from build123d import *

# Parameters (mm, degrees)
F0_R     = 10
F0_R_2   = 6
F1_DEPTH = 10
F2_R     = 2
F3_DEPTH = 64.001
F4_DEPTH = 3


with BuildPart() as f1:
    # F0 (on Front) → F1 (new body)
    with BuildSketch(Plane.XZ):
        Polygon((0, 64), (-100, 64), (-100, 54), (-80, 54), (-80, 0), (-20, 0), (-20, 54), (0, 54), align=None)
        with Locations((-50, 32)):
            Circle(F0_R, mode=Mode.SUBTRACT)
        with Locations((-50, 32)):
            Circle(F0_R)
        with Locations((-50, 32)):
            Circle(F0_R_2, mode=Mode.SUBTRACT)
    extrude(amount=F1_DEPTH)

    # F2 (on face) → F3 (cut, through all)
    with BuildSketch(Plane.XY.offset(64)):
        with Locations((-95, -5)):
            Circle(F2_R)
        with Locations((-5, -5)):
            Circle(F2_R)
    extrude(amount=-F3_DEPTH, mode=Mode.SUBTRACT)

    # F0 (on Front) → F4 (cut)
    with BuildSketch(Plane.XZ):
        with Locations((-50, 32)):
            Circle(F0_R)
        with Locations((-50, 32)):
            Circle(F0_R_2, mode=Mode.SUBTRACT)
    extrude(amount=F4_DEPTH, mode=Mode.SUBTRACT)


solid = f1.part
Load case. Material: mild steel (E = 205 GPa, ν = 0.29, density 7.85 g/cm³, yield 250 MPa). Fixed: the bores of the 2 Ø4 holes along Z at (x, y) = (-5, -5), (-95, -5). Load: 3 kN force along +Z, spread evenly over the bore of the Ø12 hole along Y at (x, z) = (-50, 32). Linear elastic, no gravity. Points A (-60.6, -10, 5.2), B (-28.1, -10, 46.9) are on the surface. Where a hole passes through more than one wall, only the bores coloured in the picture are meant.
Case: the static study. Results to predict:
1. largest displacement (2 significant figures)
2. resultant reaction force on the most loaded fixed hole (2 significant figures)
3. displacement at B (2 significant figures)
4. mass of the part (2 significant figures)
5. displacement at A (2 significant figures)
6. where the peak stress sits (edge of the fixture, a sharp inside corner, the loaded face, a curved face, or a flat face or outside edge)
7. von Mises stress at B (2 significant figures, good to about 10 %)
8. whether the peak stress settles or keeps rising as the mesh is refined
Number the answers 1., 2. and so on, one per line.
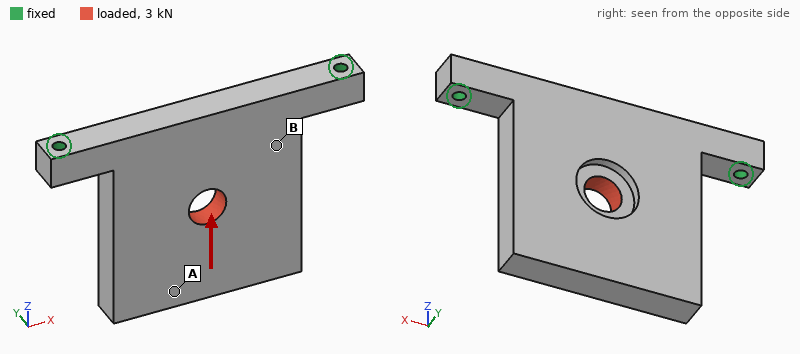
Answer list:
1. 31 µm
2. 1.7 kN
3. 13 µm
4. 320 g
5. 28 µm
6. edge of the fixture
7. 19 MPa
8. keeps rising
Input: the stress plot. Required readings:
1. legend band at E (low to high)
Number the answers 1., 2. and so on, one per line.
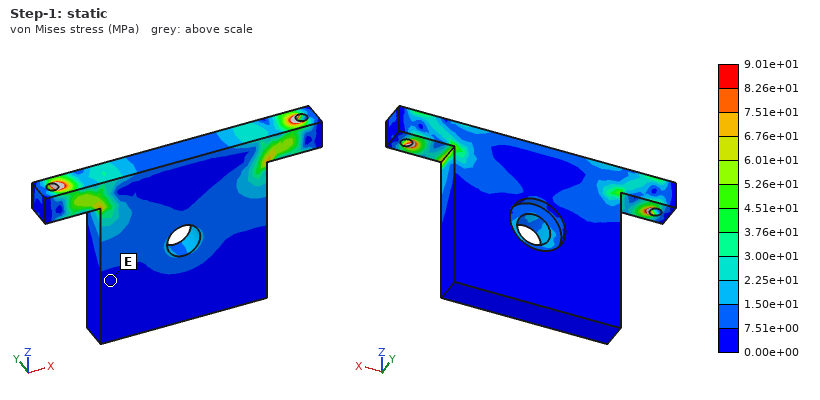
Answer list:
1. 0.00e+00 to 7.51e+00 MPa
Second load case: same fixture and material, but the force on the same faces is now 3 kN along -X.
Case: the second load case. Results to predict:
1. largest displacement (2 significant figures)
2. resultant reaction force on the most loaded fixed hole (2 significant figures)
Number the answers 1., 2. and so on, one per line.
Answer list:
1. 16 µm
2. 1.9 kN
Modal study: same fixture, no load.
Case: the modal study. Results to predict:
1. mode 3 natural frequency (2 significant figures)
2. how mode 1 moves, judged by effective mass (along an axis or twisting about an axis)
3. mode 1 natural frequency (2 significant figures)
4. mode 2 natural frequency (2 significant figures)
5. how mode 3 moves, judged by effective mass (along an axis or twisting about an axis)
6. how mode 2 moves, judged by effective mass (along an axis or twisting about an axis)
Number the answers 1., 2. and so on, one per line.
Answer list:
1. 4600 Hz
2. along Y
3. 890 Hz
4. 4100 Hz
5. along X
6. twisting about Z
